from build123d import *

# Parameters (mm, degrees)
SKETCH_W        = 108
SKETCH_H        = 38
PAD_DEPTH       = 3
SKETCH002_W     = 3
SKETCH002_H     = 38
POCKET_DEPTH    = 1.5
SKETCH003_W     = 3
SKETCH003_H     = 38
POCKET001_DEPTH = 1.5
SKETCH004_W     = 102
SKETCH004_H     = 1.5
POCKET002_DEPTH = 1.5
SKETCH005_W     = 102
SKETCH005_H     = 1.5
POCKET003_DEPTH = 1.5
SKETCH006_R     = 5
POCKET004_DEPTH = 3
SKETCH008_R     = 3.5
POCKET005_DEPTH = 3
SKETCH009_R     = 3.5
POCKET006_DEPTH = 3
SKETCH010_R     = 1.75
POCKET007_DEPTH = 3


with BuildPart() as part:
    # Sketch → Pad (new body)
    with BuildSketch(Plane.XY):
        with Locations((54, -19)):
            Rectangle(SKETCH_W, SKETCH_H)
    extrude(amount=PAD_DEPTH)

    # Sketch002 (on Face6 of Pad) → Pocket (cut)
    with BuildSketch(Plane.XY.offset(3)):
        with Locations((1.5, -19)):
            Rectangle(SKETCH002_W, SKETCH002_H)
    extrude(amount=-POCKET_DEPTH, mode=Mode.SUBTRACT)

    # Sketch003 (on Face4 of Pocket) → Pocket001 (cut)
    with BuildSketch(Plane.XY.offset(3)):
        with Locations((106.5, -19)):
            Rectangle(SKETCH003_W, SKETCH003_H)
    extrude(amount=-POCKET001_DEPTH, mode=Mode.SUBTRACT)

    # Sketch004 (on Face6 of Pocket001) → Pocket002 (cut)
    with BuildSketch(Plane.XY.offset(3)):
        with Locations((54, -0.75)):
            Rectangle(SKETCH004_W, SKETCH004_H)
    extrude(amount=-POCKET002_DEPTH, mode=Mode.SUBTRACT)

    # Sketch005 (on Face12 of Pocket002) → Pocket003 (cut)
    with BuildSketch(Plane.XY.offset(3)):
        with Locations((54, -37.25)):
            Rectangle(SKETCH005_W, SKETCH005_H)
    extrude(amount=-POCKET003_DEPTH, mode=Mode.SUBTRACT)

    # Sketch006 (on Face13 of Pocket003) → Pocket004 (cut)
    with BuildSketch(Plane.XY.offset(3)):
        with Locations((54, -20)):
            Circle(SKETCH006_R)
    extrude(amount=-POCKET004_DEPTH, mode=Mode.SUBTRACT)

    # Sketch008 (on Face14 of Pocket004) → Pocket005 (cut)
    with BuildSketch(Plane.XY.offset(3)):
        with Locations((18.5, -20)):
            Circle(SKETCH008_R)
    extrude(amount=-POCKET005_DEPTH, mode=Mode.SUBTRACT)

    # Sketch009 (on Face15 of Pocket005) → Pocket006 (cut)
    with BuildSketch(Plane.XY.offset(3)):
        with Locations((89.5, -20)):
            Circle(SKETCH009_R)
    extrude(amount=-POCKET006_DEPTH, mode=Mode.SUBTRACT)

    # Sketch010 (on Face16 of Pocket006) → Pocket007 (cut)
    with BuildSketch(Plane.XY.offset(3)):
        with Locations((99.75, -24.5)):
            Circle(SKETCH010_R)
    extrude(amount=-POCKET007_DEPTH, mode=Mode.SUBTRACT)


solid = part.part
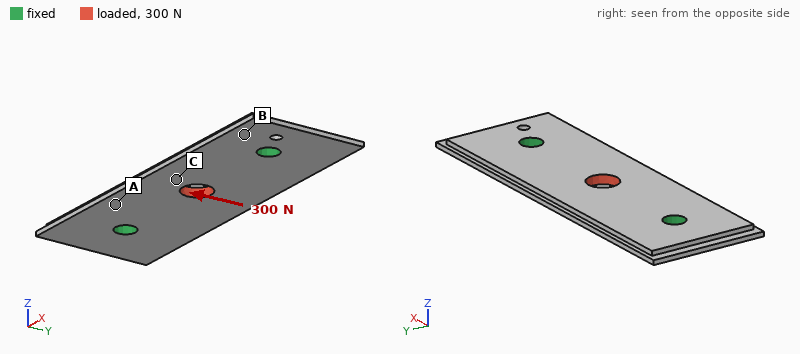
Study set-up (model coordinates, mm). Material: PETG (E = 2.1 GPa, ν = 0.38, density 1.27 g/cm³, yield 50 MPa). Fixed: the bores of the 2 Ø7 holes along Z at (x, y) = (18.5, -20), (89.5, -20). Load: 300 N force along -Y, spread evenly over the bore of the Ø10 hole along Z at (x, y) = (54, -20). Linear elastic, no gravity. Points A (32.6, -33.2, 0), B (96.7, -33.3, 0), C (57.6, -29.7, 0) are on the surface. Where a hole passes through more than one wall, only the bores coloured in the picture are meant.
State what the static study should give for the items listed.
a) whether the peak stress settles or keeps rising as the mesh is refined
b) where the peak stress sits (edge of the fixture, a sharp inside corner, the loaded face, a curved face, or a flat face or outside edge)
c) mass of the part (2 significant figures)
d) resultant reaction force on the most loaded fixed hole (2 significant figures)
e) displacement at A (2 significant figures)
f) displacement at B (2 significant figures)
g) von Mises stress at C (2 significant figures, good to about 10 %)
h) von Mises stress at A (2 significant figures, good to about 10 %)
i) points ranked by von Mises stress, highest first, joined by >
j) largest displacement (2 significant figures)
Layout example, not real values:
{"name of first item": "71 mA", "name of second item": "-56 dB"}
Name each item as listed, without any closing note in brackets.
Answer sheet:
{"whether the peak stress settles or keeps rising as the mesh is refined": "keeps rising", "where the peak stress sits": "edge of the fixture", "mass of the part": "14 g", "resultant reaction force on the most loaded fixed hole": "150 N", "displacement at A": "0.067 mm", "displacement at B": "0.034 mm", "von Mises stress at C": "3.7 MPa", "von Mises stress at A": "2.2 MPa", "points ranked by von Mises stress, highest first, joined by >": "C > A > B", "largest displacement": "0.14 mm"}
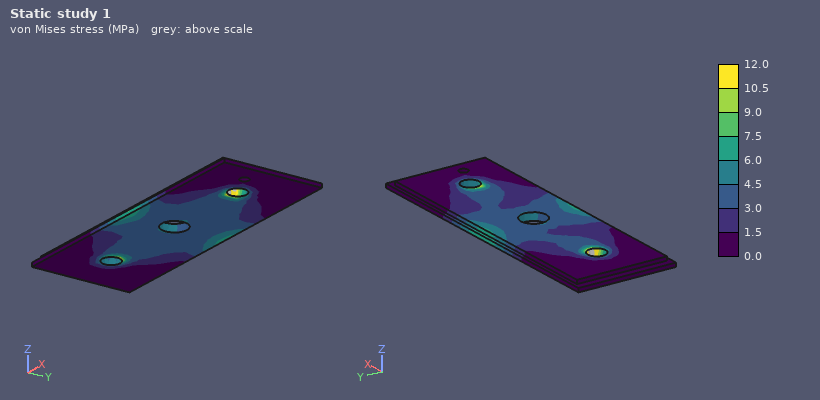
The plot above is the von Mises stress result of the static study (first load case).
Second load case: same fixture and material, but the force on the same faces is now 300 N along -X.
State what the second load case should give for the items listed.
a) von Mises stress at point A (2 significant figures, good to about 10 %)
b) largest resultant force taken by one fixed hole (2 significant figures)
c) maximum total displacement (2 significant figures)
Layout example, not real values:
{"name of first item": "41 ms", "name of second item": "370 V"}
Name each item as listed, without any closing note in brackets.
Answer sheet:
{"von Mises stress at point A": "0.97 MPa", "largest resultant force taken by one fixed hole": "150 N", "maximum total displacement": "37 µm"}
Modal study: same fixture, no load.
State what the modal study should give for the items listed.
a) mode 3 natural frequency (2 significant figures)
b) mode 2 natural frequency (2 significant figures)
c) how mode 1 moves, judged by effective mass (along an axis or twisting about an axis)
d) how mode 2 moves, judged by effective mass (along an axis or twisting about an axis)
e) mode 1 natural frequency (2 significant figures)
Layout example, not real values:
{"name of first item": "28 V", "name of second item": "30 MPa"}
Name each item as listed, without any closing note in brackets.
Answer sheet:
{"mode 3 natural frequency": "1700 Hz", "mode 2 natural frequency": "980 Hz", "how mode 1 moves, judged by effective mass": "along Z", "how mode 2 moves, judged by effective mass": "twisting about X", "mode 1 natural frequency": "800 Hz"}
